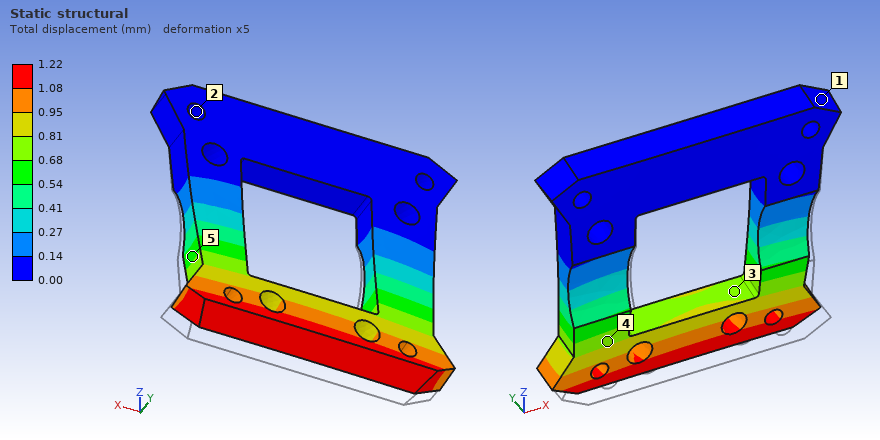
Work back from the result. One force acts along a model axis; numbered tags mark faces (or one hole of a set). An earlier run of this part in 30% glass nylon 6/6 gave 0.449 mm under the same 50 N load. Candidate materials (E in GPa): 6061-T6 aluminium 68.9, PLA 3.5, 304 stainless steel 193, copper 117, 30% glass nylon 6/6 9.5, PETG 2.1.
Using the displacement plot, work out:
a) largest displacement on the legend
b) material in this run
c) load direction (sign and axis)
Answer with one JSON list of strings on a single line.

["1.22 mm", "PLA", "+Y"]
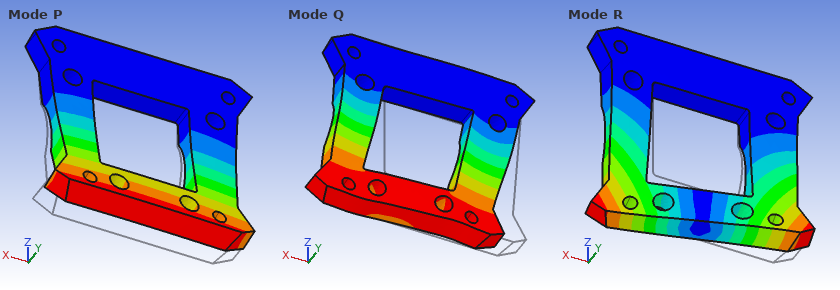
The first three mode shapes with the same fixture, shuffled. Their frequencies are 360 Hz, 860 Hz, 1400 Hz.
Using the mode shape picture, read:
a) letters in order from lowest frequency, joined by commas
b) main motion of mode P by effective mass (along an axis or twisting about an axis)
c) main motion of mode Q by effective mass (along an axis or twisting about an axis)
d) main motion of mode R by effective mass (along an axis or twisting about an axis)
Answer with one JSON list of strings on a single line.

["P, R, Q", "along Y", "along X", "twisting about Z"]
